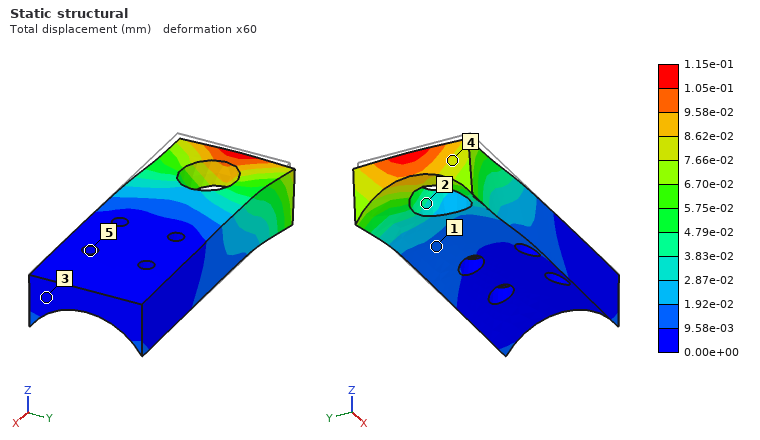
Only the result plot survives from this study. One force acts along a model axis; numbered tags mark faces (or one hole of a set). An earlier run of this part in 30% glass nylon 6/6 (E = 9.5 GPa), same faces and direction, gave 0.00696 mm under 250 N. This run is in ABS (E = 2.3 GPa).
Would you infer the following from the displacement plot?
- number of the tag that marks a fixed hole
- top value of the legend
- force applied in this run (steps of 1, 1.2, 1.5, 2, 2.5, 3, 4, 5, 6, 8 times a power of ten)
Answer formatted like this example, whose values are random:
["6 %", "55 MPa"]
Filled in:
["5", "1.15e-01 mm", "1 kN"]
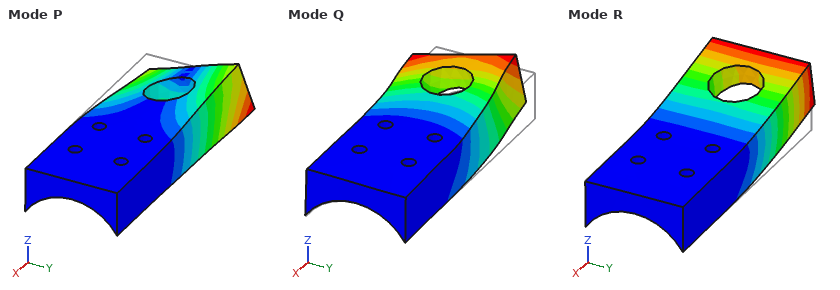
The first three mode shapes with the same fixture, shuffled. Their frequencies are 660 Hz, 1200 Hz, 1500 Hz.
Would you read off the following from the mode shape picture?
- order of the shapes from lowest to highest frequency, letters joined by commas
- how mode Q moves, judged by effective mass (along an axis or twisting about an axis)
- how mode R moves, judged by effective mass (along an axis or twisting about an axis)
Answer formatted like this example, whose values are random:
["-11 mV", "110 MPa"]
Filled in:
["R, P, Q", "along Y", "along Z"]
